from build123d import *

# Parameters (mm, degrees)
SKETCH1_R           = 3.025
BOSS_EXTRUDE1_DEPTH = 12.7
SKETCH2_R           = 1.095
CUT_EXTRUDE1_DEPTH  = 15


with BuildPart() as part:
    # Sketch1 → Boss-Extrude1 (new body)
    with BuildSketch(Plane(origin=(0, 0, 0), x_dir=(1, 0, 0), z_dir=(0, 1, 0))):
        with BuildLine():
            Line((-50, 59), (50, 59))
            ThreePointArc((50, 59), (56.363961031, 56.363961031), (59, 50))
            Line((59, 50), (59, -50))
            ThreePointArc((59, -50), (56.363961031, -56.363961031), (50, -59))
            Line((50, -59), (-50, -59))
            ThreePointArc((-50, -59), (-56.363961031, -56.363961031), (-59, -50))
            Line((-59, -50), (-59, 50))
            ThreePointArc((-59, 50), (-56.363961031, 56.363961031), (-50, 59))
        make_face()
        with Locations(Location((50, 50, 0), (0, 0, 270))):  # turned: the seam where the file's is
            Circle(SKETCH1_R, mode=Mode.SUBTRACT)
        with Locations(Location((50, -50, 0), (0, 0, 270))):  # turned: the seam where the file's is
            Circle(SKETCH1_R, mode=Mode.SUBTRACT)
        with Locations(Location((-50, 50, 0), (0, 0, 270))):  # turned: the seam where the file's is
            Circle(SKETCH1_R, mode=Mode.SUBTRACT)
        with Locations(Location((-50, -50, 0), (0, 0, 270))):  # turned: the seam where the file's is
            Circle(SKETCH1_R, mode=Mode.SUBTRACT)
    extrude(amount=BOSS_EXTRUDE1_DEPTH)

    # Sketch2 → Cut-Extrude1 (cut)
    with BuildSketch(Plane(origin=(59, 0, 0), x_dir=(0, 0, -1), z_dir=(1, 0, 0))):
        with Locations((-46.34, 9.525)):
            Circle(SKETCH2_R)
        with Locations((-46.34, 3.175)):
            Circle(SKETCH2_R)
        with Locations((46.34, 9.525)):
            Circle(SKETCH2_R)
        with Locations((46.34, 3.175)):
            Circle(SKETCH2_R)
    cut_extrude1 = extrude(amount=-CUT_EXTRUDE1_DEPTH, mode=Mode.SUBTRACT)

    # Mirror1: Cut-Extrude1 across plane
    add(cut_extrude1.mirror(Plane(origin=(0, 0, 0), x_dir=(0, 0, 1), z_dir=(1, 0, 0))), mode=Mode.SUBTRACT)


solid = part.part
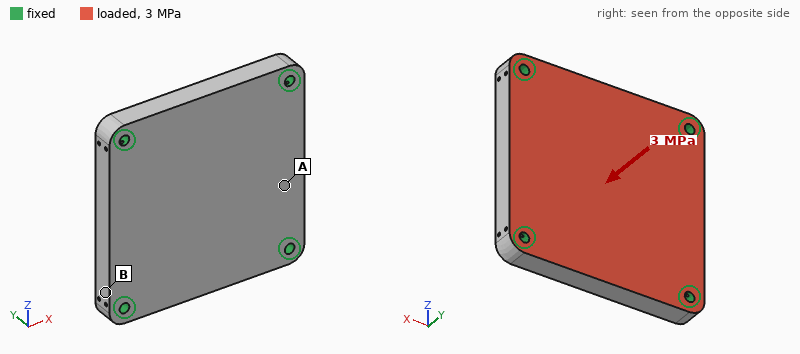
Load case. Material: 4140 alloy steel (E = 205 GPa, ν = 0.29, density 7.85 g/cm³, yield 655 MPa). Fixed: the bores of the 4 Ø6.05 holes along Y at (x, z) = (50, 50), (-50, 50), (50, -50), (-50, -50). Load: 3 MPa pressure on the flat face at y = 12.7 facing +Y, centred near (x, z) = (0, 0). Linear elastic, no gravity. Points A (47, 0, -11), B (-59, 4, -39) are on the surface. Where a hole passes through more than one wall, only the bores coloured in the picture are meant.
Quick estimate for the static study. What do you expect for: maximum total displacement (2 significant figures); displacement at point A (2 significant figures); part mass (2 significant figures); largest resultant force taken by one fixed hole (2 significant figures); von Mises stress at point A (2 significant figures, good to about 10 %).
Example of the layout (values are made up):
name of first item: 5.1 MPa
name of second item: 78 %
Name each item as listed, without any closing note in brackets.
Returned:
maximum total displacement: 79 µm
displacement at point A: 47 µm
part mass: 1.4 kg
largest resultant force taken by one fixed hole: 10 kN
von Mises stress at point A: 62 MPa
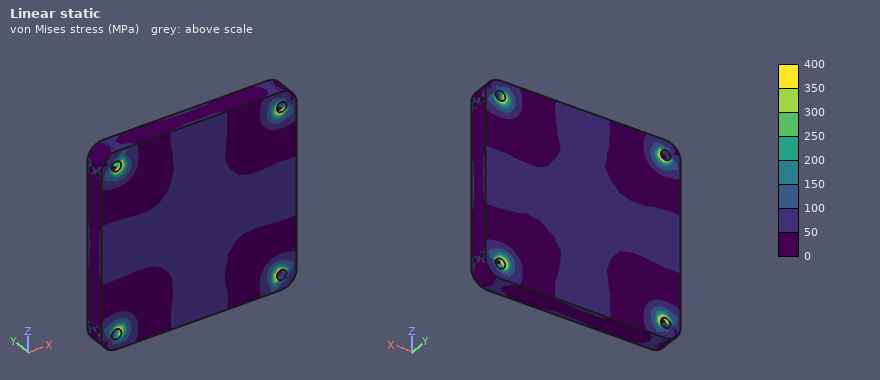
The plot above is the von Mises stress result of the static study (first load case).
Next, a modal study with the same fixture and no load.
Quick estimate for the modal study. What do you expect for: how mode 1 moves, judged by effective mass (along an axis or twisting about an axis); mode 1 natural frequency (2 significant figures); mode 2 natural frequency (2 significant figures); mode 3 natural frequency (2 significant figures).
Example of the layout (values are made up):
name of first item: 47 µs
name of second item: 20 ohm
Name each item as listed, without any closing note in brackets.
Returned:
how mode 1 moves, judged by effective mass: along Y
mode 1 natural frequency: 3700 Hz
mode 2 natural frequency: 6200 Hz
mode 3 natural frequency: 6300 Hz
